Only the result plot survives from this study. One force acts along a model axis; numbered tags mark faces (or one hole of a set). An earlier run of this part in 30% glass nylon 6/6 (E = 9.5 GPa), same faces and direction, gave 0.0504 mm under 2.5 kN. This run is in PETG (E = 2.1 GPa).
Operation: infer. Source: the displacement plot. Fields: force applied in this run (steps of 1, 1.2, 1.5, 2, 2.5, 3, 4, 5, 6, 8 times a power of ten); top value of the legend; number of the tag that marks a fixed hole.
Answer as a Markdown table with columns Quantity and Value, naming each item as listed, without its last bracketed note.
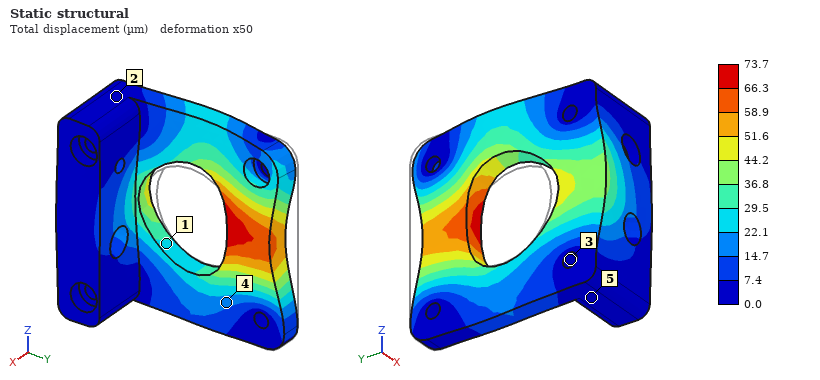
| Quantity | Value |
|---|---|
| force applied in this run | 800 N |
| top value of the legend | 73.7 µm |
| number of the tag that marks a fixed hole | 3 |
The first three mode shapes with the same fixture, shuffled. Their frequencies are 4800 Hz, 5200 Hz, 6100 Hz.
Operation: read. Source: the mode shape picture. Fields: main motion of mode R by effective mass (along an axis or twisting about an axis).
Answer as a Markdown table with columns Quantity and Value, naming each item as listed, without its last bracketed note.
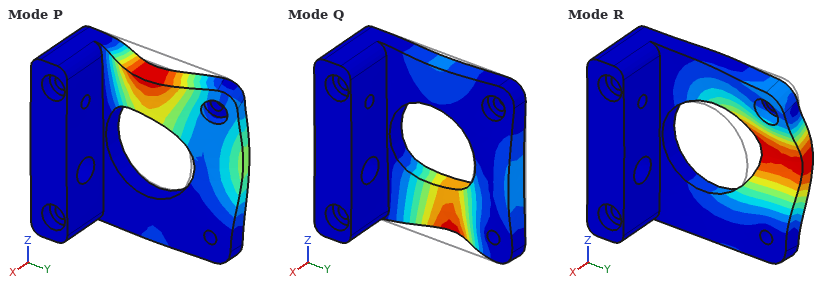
| Quantity | Value |
|---|---|
| main motion of mode R by effective mass | along X |
